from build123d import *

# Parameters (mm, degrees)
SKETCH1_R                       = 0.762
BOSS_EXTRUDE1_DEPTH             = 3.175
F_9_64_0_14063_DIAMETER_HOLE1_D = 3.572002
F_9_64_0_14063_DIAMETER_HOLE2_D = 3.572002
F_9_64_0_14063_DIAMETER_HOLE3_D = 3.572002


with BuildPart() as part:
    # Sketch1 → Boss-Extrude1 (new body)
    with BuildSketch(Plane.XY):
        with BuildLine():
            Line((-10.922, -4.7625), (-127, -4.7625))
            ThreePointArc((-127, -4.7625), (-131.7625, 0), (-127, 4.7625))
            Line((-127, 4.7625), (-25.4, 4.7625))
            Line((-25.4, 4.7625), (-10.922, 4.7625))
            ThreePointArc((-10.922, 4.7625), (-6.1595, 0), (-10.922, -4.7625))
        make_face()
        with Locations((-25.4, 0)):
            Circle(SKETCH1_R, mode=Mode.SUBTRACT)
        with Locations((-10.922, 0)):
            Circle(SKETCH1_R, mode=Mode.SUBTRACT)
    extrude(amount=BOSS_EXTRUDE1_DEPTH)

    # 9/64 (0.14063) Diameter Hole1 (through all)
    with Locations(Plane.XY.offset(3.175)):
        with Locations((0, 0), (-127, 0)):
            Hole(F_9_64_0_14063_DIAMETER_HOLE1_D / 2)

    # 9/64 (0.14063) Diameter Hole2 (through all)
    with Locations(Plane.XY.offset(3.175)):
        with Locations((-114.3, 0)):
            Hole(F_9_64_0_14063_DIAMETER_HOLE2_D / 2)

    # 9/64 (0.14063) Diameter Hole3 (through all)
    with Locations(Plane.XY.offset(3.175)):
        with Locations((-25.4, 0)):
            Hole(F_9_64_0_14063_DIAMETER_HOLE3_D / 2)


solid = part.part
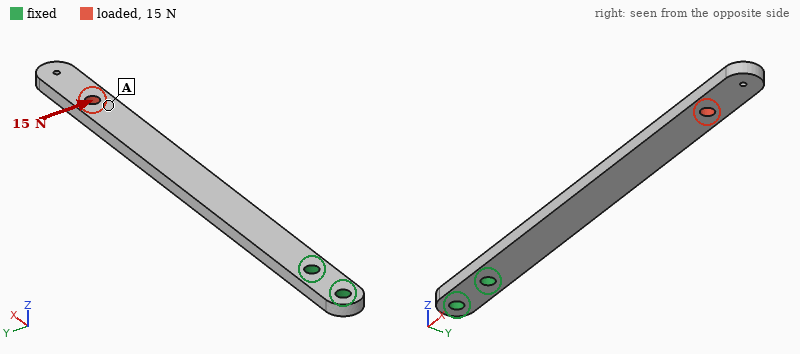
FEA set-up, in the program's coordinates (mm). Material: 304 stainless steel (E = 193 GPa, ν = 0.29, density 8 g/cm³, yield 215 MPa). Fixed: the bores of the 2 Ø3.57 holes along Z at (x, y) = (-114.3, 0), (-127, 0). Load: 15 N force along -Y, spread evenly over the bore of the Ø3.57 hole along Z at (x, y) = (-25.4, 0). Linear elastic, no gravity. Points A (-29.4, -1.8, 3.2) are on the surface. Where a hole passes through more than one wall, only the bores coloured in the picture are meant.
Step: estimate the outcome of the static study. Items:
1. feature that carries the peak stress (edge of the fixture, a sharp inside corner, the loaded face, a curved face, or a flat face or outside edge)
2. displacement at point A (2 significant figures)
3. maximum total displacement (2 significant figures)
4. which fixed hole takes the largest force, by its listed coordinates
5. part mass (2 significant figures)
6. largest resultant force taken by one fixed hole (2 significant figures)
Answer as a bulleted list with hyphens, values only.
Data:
- edge of the fixture
- 0.080 mm
- 0.11 mm
- (-114.3, 0)
- 29 g
- 55 N
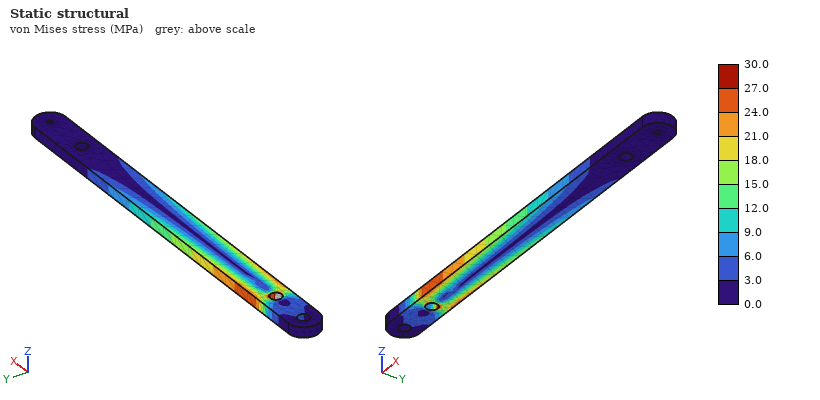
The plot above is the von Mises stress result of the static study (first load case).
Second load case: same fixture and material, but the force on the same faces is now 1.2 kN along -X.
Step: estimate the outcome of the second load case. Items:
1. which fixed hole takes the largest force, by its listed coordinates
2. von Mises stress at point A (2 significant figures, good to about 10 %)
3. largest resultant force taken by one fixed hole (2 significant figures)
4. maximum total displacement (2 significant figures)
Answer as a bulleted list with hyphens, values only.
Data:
- (-114.3, 0)
- 43 MPa
- 1.1 kN
- 19 µm
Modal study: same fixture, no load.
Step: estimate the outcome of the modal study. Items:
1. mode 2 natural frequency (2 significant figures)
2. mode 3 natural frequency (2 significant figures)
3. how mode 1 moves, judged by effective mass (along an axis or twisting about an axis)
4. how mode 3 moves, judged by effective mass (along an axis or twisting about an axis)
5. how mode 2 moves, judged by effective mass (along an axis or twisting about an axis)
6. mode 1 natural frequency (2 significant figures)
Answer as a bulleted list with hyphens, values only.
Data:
- 640 Hz
- 1400 Hz
- along Z
- along Z
- along Y
- 230 Hz
